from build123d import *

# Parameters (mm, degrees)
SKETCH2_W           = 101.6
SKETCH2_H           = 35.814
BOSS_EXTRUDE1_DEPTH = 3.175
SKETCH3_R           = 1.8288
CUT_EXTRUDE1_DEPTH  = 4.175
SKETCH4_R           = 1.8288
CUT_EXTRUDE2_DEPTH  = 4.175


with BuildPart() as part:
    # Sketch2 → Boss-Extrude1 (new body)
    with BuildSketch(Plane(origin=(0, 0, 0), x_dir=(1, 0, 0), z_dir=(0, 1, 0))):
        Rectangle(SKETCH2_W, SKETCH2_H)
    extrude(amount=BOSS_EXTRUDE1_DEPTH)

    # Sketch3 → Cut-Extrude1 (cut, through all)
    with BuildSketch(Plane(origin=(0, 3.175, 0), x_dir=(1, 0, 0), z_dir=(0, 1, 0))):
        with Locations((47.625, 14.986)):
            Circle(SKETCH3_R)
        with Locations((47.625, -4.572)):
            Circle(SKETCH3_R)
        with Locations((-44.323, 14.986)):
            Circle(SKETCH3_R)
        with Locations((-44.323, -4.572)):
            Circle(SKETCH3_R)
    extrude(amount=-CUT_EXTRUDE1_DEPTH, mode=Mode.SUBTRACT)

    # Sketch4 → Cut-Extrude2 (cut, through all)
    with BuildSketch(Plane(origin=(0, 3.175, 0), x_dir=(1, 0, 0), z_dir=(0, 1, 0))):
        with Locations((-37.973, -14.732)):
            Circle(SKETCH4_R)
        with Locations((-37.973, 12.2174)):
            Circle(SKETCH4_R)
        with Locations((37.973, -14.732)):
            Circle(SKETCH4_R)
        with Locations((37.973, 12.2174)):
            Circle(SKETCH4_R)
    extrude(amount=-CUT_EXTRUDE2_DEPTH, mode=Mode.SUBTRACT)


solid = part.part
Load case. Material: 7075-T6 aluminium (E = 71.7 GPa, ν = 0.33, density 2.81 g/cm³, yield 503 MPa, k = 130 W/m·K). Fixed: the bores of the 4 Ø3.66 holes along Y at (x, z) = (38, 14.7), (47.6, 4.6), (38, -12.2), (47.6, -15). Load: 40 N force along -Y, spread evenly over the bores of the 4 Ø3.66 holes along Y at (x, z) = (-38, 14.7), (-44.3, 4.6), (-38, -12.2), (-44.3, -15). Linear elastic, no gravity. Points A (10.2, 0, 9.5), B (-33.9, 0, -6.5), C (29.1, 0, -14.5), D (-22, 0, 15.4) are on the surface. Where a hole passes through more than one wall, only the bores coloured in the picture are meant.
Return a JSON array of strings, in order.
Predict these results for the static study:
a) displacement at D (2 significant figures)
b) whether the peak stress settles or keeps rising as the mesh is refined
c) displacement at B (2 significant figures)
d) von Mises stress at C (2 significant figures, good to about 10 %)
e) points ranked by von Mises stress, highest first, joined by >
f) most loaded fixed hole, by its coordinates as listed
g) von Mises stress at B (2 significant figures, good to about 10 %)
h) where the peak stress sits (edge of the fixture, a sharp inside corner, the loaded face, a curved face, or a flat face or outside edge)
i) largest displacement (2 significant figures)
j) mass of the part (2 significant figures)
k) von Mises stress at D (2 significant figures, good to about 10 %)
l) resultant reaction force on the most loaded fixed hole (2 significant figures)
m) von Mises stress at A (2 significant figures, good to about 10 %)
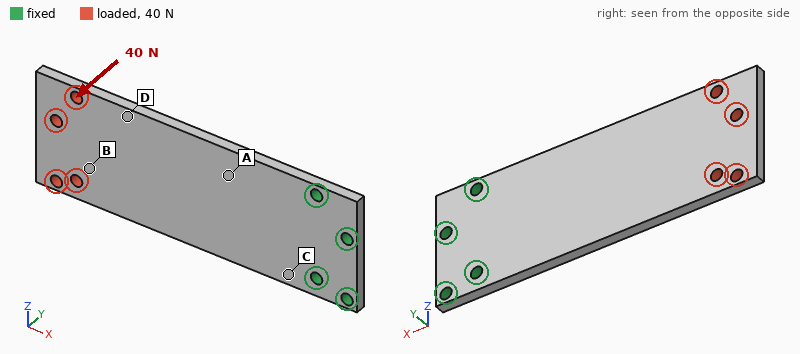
["0.61 mm", "keeps rising", "0.83 mm", "49 MPa", "C > A > D > B", "(38, -12.2)", "5.9 MPa", "edge of the fixture", "1.1 mm", "32 g", "13 MPa", "88 N", "34 MPa"]
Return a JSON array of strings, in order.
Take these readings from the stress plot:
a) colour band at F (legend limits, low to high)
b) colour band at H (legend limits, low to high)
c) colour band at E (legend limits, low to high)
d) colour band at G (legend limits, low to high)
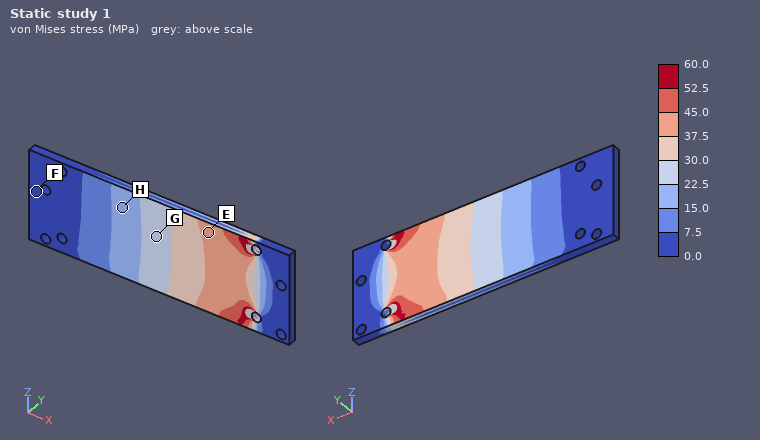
["0.0 to 7.5 MPa", "15.0 to 22.5 MPa", "37.5 to 45.0 MPa", "22.5 to 30.0 MPa"]
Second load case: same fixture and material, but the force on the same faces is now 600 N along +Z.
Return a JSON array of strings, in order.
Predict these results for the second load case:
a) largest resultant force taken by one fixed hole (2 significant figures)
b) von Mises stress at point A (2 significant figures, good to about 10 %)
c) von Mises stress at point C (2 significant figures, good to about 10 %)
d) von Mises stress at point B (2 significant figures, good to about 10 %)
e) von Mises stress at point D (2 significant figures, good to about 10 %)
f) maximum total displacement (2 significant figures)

["1.6 kN", "26 MPa", "50 MPa", "11 MPa", "15 MPa", "0.16 mm"]
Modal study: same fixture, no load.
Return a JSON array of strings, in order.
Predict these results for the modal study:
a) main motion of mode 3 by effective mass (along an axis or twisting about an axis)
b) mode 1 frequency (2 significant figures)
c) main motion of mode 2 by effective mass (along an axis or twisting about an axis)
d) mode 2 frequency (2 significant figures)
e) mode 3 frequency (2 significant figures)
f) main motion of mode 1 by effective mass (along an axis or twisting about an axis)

["along Y", "340 Hz", "twisting about X", "1700 Hz", "2100 Hz", "along Y"]
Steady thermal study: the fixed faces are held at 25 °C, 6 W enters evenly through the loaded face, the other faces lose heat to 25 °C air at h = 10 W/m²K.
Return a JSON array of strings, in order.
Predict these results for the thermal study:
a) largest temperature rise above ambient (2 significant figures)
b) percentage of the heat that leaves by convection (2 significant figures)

["31 K", "18 %"]
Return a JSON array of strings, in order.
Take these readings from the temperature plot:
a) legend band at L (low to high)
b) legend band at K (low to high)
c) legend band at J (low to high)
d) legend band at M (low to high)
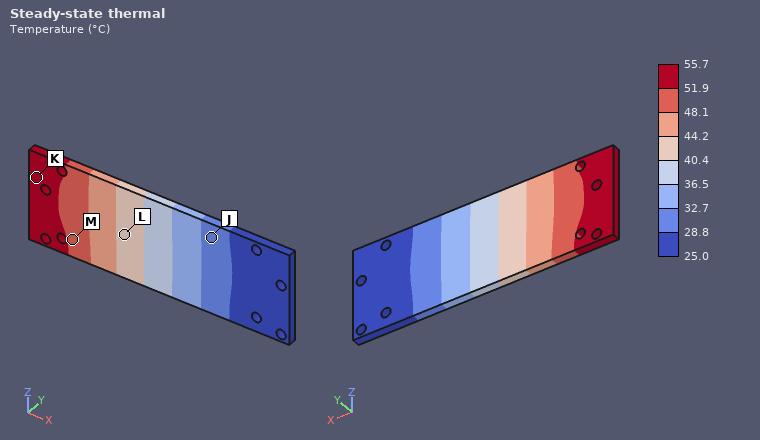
["40.4 to 44.2 °C", "51.9 to 55.7 °C", "28.8 to 32.7 °C", "48.1 to 51.9 °C"]
